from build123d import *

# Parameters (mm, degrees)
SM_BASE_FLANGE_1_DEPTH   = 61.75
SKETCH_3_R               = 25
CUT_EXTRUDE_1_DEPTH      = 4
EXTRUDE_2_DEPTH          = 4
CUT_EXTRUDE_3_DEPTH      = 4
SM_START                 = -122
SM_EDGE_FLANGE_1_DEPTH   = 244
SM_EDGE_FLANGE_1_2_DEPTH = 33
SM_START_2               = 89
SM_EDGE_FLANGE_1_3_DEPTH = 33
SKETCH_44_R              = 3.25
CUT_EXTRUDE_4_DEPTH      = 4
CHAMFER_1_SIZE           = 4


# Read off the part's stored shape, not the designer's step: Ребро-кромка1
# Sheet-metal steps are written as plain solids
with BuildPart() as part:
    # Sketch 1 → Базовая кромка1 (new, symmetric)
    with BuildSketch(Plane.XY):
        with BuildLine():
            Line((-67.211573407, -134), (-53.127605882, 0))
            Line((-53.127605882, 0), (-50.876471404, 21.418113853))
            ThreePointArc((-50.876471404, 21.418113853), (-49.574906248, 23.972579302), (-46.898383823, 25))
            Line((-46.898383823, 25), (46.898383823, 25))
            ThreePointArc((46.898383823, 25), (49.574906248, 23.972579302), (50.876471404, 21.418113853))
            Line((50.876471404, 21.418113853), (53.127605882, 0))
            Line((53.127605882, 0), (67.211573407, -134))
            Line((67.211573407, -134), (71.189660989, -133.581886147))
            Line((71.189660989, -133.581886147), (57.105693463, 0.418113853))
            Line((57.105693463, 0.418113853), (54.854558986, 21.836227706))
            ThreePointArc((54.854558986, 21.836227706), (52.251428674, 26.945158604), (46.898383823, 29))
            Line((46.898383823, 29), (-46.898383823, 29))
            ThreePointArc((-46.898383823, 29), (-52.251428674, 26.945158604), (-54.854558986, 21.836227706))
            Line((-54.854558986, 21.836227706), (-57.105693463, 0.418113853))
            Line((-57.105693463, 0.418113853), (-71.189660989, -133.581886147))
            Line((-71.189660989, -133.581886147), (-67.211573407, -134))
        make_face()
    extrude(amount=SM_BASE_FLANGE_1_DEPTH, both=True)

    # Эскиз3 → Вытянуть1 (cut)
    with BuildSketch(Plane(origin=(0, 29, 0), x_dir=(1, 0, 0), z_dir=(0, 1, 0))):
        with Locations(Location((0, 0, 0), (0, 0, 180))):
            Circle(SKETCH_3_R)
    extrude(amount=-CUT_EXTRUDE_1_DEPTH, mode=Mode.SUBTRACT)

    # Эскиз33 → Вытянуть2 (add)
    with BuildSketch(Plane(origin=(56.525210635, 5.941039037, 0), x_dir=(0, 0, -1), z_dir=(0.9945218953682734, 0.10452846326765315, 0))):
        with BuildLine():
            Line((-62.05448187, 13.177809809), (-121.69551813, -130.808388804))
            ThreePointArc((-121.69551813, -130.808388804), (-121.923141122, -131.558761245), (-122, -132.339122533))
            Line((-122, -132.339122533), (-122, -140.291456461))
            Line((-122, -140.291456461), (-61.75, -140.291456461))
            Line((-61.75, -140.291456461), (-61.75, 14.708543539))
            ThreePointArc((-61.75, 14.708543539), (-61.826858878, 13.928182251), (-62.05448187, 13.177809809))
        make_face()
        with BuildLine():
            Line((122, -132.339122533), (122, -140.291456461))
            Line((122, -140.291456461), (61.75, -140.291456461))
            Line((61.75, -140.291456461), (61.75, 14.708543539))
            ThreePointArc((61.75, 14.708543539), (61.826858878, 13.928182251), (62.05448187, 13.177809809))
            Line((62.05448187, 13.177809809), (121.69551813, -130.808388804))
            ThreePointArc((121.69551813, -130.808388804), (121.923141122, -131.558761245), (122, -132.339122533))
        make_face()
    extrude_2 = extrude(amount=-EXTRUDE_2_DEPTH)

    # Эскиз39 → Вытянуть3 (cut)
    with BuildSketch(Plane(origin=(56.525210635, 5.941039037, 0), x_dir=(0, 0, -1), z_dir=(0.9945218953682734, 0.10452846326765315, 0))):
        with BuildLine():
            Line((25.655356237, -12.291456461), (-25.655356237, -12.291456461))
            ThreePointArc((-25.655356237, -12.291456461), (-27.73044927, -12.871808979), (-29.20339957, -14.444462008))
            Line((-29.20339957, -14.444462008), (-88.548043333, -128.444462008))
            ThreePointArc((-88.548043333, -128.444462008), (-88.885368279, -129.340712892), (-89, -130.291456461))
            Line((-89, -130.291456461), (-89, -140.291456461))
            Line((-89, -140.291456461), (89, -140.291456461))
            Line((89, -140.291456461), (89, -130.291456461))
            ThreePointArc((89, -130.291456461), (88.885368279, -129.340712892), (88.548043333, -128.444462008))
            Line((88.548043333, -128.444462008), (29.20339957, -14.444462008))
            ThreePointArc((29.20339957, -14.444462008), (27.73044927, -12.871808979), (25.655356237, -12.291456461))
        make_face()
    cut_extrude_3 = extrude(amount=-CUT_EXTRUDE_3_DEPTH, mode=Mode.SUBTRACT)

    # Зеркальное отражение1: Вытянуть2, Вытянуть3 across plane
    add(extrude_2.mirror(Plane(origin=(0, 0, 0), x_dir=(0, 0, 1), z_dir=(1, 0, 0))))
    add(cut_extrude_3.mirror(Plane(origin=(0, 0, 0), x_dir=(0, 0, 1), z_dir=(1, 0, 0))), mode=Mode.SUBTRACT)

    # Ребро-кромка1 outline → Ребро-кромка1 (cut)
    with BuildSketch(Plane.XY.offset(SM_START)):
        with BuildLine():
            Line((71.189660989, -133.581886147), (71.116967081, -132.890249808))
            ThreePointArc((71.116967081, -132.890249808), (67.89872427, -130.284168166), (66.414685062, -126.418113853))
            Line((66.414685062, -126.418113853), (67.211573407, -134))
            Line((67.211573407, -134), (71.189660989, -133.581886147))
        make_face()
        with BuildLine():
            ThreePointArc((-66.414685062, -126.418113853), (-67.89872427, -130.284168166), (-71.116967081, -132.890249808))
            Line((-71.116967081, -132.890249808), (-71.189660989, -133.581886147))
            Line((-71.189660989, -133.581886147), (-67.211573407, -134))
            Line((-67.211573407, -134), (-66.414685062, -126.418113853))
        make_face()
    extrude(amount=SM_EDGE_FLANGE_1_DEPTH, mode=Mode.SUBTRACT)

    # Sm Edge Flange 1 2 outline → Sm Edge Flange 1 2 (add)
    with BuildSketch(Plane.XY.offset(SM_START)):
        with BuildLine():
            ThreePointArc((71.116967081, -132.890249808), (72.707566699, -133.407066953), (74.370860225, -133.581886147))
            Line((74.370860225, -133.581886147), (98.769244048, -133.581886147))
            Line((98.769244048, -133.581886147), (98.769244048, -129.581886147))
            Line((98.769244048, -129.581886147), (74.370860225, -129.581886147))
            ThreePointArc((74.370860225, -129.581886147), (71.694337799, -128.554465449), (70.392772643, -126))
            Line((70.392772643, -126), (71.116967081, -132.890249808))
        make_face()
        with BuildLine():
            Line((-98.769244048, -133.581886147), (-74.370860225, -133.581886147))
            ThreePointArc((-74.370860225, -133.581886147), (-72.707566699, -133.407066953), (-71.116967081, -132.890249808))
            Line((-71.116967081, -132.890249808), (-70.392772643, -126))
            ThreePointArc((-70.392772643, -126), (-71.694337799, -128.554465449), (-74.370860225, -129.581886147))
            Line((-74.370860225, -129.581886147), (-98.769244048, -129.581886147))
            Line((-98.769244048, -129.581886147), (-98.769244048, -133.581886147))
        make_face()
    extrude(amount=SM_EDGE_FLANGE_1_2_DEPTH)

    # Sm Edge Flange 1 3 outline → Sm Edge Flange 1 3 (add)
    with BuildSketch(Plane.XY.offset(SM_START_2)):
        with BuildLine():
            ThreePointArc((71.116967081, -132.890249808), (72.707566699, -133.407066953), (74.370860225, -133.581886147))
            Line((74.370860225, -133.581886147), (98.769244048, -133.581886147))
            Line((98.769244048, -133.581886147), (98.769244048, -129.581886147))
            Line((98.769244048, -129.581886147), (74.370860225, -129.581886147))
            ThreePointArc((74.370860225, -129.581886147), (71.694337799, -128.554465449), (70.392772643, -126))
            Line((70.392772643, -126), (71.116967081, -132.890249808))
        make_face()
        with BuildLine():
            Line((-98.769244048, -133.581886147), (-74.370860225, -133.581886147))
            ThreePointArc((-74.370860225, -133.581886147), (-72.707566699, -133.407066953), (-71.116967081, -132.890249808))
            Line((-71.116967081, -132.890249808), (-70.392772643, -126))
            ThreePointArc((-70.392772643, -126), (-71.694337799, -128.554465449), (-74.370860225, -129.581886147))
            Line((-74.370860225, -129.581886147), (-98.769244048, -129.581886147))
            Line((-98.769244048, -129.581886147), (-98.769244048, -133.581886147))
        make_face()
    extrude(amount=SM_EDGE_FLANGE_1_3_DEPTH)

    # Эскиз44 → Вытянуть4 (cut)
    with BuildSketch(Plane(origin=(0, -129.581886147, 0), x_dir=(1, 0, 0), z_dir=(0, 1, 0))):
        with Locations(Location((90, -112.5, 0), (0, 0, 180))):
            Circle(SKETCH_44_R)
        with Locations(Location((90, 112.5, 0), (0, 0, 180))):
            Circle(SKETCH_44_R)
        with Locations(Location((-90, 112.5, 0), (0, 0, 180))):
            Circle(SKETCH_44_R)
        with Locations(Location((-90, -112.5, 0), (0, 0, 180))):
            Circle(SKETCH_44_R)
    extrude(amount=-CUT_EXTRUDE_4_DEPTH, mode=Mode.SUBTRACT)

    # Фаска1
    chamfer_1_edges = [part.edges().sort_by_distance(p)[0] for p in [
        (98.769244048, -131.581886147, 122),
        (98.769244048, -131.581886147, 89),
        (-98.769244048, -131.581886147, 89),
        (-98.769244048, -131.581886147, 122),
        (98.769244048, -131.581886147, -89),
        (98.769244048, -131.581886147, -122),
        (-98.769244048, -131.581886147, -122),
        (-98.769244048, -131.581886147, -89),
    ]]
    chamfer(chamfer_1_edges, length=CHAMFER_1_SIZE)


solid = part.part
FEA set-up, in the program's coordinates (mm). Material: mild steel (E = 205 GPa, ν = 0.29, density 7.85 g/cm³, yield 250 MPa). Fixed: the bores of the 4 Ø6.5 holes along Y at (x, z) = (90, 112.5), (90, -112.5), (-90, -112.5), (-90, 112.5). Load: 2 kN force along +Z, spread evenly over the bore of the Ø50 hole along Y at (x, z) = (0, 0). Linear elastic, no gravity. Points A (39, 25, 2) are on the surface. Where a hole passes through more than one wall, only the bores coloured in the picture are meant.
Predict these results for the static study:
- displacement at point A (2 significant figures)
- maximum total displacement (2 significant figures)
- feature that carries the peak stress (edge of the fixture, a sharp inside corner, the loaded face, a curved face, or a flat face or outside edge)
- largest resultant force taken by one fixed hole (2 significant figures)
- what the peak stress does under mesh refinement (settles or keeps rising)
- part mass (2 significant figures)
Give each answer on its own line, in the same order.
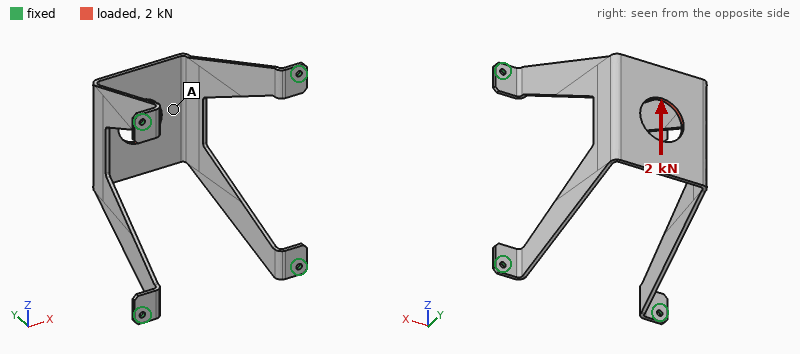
0.10 mm
0.11 mm
edge of the fixture
860 N
keeps rising
1.3 kg
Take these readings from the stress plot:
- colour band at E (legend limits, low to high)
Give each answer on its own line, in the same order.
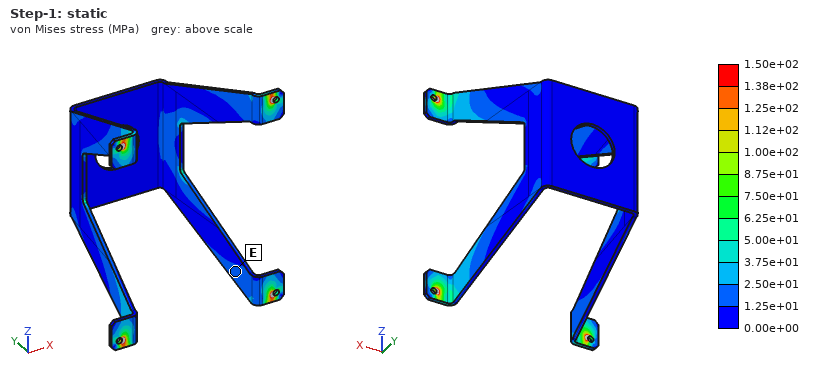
1.25e+01 to 2.50e+01 MPa
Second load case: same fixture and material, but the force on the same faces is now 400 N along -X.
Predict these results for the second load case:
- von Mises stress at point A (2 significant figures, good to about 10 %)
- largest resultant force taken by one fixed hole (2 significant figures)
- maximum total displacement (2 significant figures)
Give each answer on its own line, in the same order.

20 MPa
190 N
0.94 mm
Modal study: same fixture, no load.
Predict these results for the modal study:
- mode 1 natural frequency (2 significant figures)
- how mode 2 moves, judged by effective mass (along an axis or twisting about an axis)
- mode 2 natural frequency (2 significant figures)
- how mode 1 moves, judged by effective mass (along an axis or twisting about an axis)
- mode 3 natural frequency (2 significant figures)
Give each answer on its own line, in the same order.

120 Hz
twisting about Y
450 Hz
along X
490 Hz
